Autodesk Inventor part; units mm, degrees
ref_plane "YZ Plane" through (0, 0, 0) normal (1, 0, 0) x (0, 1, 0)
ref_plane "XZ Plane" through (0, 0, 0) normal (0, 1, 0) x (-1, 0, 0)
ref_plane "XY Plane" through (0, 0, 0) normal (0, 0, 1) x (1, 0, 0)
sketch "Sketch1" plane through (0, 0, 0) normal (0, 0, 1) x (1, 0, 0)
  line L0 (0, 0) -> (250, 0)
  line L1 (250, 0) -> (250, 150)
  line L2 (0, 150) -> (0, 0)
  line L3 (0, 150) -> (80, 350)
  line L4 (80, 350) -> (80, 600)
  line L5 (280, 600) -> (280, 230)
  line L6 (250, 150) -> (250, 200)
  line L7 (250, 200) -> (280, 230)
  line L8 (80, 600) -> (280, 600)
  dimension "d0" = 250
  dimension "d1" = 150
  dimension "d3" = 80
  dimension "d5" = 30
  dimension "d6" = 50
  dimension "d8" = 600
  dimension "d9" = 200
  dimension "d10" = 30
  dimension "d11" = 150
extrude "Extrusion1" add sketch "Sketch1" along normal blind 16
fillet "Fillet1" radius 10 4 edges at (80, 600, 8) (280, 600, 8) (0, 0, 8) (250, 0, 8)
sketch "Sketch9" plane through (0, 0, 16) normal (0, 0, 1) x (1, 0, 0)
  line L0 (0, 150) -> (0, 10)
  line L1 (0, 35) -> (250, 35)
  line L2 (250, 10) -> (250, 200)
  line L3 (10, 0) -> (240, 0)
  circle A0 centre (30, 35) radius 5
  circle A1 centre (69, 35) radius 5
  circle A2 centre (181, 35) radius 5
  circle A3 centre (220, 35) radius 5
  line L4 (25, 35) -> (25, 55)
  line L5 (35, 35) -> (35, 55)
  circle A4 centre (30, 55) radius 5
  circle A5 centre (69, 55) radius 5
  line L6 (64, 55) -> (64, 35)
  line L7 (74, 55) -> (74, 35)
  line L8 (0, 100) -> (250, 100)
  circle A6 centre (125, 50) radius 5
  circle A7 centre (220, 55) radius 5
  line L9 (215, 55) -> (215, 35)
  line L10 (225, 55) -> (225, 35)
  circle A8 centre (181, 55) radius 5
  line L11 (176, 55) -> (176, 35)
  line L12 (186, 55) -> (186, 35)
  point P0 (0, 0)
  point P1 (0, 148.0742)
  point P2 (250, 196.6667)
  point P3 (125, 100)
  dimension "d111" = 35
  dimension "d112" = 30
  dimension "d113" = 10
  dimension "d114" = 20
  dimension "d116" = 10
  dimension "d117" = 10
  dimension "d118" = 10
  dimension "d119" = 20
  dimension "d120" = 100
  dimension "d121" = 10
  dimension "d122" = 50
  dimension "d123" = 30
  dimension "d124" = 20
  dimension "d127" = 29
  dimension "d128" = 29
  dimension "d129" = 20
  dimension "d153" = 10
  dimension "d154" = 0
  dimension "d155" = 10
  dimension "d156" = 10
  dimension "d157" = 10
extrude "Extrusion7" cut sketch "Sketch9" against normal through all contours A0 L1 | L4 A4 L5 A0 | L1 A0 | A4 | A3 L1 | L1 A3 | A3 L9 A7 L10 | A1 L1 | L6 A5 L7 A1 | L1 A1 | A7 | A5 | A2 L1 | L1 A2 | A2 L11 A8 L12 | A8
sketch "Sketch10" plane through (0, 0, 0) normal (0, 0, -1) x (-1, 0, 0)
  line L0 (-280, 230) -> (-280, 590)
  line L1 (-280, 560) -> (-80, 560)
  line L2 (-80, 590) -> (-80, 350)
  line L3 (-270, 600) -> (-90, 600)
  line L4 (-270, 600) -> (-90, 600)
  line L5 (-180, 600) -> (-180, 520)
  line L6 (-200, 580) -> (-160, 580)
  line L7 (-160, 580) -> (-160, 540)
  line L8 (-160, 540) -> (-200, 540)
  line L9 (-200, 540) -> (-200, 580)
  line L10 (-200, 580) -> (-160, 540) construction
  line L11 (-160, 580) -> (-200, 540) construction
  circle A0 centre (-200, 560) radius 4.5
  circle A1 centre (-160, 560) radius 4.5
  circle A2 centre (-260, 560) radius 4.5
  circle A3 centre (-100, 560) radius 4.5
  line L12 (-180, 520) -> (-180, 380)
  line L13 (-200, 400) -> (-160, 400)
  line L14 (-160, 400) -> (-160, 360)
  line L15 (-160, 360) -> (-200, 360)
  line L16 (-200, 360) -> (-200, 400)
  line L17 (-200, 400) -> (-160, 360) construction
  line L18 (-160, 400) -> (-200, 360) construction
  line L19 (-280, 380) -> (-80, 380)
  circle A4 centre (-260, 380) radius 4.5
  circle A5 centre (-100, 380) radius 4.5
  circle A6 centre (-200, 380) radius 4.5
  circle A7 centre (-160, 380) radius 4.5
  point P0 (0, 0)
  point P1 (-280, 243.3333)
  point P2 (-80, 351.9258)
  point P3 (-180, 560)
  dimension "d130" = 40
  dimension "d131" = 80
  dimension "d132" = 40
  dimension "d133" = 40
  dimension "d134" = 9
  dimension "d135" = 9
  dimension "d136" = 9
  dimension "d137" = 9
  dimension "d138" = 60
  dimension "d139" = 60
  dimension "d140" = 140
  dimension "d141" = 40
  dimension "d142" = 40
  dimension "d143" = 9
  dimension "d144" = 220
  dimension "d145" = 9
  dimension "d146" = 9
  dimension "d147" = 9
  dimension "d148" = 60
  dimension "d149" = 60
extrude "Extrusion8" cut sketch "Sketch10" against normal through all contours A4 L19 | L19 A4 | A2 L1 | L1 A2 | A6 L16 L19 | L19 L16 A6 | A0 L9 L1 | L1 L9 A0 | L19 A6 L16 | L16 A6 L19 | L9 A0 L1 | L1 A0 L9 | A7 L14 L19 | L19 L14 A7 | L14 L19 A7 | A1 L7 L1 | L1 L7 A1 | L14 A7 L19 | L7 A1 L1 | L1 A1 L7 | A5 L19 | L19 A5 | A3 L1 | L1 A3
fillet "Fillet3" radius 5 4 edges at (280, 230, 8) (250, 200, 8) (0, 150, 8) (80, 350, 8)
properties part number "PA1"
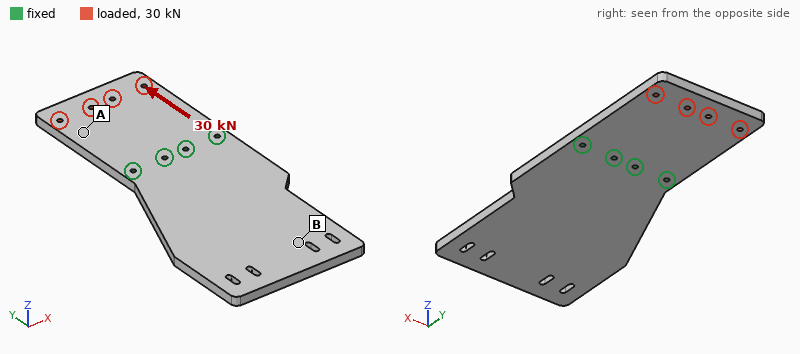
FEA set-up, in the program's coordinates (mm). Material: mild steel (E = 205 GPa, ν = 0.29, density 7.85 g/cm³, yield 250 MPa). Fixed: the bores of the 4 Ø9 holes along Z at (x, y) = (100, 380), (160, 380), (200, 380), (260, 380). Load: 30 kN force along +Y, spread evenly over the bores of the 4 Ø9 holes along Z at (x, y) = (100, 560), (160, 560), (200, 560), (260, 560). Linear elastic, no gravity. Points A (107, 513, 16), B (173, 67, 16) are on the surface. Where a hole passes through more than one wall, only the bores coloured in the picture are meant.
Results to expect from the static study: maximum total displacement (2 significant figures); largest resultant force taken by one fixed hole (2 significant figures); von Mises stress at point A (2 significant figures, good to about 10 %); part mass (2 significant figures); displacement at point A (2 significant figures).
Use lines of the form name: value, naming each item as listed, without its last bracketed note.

maximum total displacement: 9.7 µm
largest resultant force taken by one fixed hole: 7.9 kN
von Mises stress at point A: 9.1 MPa
part mass: 17 kg
displacement at point A: 6.5 µm
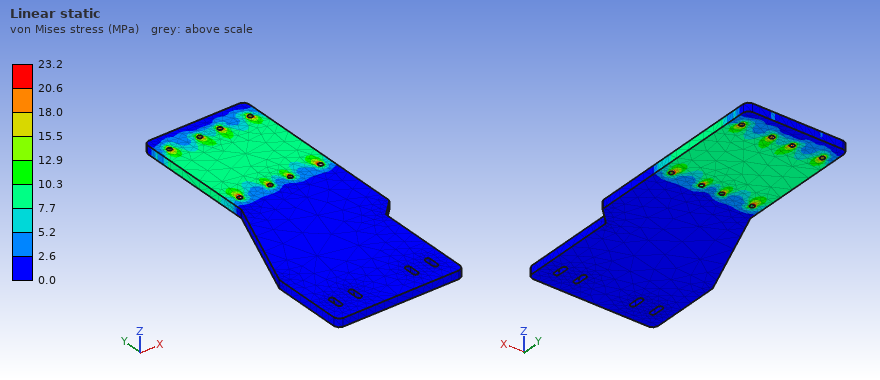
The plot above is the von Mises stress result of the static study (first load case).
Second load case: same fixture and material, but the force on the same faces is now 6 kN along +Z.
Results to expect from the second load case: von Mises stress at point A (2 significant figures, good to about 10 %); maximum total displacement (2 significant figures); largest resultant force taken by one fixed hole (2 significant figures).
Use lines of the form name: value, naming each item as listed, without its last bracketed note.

von Mises stress at point A: 34 MPa
maximum total displacement: 1.1 mm
largest resultant force taken by one fixed hole: 2.6 kN
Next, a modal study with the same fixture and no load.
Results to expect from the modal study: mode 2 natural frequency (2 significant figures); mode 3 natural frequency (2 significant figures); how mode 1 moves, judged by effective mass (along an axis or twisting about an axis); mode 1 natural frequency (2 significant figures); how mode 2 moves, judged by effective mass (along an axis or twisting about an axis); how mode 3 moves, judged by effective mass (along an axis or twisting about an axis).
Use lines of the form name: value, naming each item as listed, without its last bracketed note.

mode 2 natural frequency: 270 Hz
mode 3 natural frequency: 290 Hz
how mode 1 moves, judged by effective mass: along Z
mode 1 natural frequency: 84 Hz
how mode 2 moves, judged by effective mass: along Z
how mode 3 moves, judged by effective mass: twisting about Y
